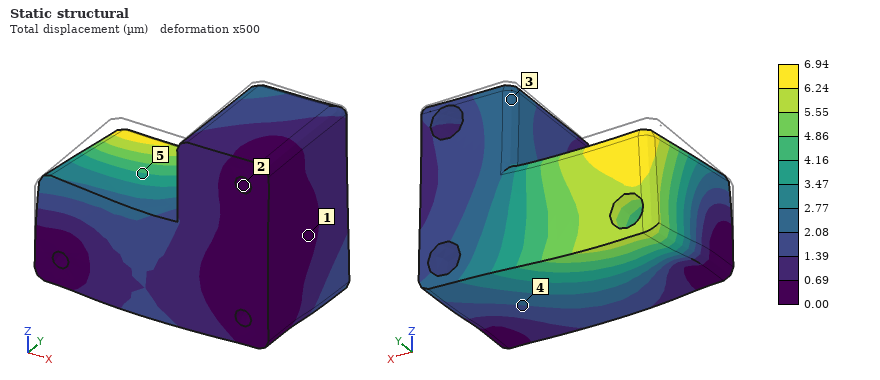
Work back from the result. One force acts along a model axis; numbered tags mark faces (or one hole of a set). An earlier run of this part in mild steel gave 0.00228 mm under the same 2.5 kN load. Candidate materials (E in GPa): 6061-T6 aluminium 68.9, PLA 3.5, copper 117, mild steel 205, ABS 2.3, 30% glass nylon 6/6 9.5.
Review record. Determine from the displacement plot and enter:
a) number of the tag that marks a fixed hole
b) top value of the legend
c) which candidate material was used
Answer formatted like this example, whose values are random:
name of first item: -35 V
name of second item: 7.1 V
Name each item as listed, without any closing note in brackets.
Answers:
number of the tag that marks a fixed hole: 2
top value of the legend: 6.94 µm
which candidate material was used: 6061-T6 aluminium
